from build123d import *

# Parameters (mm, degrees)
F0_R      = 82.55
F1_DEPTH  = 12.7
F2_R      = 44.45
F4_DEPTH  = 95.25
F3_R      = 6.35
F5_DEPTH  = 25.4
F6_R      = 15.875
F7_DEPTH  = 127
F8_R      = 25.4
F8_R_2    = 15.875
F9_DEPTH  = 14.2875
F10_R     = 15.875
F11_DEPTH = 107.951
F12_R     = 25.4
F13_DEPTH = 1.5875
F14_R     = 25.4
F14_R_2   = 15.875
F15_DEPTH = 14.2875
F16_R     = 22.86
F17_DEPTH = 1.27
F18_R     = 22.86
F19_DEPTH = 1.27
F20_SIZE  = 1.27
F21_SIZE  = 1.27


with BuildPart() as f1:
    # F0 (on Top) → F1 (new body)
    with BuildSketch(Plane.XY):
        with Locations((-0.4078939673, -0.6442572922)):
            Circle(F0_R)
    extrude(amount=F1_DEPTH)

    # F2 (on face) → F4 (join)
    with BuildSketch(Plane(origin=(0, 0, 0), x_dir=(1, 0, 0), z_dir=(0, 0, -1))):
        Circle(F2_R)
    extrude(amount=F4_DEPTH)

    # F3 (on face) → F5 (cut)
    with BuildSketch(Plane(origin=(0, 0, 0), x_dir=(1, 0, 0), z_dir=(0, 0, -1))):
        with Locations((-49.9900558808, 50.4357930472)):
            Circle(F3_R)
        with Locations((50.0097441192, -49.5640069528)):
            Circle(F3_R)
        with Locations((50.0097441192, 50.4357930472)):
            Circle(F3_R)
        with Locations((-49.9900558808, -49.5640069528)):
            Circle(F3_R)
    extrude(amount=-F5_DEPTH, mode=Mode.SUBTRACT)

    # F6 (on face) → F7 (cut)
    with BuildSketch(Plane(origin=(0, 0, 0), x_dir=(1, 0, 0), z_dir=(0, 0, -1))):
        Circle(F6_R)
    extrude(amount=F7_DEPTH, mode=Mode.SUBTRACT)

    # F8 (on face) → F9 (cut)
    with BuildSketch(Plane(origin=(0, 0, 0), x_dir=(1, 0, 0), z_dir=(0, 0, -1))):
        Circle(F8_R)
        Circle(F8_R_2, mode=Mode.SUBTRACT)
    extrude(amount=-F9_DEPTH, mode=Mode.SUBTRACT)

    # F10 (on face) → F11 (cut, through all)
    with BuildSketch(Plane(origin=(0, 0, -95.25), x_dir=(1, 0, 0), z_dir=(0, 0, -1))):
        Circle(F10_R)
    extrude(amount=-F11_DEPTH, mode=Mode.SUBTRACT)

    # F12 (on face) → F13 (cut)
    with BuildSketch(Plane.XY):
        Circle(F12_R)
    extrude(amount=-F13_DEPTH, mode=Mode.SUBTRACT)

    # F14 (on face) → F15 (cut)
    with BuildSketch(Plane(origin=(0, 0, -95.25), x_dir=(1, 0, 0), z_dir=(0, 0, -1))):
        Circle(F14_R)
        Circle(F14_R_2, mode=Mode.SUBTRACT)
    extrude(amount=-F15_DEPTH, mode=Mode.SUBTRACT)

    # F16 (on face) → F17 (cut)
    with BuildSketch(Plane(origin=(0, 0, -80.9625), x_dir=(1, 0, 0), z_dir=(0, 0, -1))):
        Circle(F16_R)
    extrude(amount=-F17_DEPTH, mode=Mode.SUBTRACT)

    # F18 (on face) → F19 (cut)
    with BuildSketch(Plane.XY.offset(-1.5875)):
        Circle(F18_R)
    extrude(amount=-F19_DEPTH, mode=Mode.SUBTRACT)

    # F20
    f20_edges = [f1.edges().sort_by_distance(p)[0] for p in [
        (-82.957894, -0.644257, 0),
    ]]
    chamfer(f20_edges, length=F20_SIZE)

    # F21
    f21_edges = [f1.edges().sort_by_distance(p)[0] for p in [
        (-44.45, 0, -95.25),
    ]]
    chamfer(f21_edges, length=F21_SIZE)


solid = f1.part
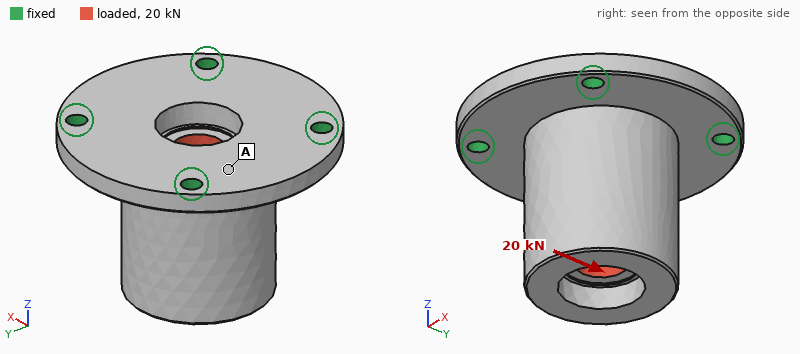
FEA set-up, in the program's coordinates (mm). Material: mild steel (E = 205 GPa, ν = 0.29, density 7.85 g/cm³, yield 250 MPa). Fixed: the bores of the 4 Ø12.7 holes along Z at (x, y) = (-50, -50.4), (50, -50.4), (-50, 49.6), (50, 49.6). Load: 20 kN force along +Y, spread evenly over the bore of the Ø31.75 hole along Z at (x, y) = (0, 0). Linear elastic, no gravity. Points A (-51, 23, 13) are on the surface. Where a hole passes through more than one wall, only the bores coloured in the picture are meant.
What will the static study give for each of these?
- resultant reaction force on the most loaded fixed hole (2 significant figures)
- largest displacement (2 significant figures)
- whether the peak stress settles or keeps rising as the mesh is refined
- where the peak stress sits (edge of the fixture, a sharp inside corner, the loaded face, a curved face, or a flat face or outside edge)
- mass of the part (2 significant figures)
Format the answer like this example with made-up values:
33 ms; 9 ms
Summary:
7.6 kN; 38 µm; keeps rising; edge of the fixture; 5.8 kg
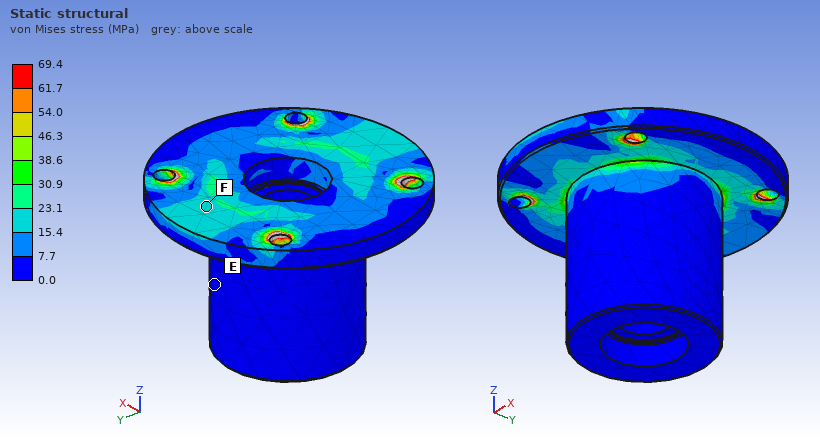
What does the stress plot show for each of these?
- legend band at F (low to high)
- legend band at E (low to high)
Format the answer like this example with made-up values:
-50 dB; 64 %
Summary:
15.4 to 23.1 MPa; 0.0 to 7.7 MPa
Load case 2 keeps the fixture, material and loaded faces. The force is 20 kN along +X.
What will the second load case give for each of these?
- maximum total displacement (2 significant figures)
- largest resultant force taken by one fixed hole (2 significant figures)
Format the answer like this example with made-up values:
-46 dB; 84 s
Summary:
39 µm; 7.7 kN
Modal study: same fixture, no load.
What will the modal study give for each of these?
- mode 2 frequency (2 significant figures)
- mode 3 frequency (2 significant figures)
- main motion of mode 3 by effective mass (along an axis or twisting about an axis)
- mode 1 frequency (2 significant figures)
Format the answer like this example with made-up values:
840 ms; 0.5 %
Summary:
2000 Hz; 3100 Hz; along Z; 2000 Hz
